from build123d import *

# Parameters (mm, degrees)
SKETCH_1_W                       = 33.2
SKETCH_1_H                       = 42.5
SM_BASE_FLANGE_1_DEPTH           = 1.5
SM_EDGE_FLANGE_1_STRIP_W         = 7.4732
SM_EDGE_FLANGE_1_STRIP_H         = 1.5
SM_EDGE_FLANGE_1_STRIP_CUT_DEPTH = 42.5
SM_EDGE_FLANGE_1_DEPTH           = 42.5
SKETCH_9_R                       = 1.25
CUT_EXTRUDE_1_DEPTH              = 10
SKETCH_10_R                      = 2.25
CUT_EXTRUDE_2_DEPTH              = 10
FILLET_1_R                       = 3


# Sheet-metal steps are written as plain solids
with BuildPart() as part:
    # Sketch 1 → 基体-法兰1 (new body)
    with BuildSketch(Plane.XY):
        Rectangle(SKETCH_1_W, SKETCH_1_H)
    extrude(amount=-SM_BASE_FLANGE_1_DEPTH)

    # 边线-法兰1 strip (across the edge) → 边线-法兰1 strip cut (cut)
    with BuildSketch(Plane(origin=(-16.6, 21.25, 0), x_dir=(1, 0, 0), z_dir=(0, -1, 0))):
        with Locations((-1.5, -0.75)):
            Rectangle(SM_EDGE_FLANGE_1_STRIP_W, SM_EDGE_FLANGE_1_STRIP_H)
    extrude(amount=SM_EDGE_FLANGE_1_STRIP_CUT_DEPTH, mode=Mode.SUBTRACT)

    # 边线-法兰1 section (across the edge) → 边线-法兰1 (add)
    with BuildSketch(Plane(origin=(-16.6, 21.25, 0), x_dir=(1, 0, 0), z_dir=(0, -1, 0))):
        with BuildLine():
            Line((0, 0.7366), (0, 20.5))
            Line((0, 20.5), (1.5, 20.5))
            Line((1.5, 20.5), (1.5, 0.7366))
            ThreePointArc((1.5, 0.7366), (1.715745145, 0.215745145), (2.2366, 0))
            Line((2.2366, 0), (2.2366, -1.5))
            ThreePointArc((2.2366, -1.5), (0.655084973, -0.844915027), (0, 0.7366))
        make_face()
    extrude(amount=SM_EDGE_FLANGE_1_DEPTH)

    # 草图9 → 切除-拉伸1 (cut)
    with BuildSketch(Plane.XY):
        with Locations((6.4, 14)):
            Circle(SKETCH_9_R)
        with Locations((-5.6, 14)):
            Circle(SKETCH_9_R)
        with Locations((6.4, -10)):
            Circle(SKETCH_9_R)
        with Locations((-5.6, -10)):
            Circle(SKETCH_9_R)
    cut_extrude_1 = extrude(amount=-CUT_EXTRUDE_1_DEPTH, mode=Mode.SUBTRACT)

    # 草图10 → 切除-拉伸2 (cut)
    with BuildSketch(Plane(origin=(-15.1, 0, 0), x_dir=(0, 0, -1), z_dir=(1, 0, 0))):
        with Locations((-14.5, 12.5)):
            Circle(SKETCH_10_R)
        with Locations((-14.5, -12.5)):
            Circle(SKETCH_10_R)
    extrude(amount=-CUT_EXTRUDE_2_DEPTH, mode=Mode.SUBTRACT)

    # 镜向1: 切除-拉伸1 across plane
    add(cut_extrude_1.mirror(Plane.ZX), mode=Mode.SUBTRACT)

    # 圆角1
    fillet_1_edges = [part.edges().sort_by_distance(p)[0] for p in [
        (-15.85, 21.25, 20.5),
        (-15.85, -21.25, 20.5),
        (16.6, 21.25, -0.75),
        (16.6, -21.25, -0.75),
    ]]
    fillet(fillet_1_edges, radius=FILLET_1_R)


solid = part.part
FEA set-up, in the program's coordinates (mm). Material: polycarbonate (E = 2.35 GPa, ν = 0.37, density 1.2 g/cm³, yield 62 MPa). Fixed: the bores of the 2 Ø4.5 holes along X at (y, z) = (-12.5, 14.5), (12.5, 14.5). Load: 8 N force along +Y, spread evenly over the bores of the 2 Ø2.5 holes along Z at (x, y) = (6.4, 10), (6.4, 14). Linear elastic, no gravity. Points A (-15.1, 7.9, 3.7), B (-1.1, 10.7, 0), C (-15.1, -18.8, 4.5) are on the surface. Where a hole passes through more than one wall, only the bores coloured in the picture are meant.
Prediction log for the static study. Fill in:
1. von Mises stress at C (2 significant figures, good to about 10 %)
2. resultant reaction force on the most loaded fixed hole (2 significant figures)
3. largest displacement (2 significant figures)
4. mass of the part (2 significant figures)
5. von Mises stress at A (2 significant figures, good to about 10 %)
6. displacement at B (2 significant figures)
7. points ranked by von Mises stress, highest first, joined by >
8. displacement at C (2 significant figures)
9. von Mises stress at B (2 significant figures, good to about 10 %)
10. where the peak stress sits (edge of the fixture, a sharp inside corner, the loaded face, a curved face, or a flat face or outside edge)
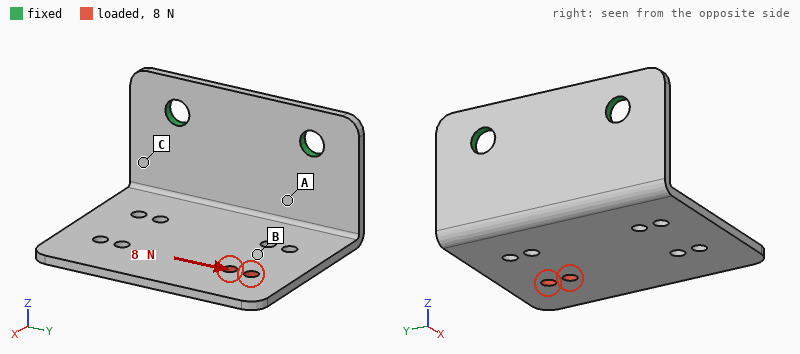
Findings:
2.7 MPa
8.5 N
0.70 mm
3.9 g
3.8 MPa
0.33 mm
A > C > B
0.18 mm
1.2 MPa
a flat face or outside edge
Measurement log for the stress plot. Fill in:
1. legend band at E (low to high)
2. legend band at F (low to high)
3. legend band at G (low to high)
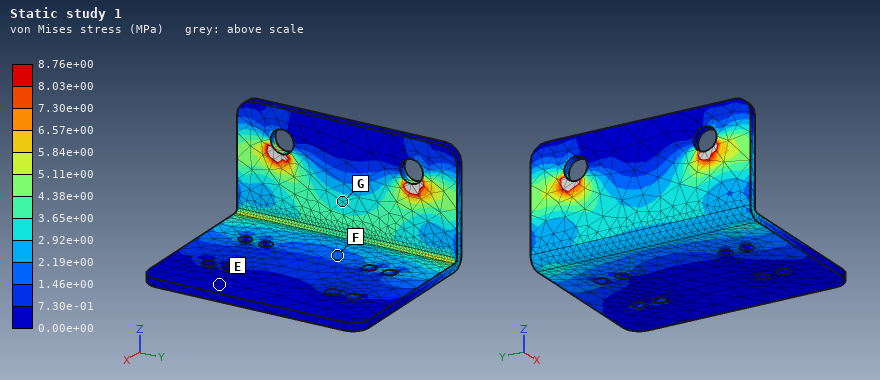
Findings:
0.00e+00 to 7.30e-01 MPa
1.46e+00 to 2.19e+00 MPa
2.92e+00 to 3.65e+00 MPa
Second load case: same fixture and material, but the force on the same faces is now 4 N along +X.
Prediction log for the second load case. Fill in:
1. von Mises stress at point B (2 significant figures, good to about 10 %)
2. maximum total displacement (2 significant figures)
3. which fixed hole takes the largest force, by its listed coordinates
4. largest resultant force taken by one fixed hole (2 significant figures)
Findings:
0.31 MPa
0.59 mm
(12.5, 14.5)
3.7 N
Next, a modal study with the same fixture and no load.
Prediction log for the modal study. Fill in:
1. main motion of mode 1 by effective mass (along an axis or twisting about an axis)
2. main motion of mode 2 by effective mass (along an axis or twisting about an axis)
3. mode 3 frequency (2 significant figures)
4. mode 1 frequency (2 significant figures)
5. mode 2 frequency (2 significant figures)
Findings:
along Z
along Y
660 Hz
200 Hz
420 Hz
